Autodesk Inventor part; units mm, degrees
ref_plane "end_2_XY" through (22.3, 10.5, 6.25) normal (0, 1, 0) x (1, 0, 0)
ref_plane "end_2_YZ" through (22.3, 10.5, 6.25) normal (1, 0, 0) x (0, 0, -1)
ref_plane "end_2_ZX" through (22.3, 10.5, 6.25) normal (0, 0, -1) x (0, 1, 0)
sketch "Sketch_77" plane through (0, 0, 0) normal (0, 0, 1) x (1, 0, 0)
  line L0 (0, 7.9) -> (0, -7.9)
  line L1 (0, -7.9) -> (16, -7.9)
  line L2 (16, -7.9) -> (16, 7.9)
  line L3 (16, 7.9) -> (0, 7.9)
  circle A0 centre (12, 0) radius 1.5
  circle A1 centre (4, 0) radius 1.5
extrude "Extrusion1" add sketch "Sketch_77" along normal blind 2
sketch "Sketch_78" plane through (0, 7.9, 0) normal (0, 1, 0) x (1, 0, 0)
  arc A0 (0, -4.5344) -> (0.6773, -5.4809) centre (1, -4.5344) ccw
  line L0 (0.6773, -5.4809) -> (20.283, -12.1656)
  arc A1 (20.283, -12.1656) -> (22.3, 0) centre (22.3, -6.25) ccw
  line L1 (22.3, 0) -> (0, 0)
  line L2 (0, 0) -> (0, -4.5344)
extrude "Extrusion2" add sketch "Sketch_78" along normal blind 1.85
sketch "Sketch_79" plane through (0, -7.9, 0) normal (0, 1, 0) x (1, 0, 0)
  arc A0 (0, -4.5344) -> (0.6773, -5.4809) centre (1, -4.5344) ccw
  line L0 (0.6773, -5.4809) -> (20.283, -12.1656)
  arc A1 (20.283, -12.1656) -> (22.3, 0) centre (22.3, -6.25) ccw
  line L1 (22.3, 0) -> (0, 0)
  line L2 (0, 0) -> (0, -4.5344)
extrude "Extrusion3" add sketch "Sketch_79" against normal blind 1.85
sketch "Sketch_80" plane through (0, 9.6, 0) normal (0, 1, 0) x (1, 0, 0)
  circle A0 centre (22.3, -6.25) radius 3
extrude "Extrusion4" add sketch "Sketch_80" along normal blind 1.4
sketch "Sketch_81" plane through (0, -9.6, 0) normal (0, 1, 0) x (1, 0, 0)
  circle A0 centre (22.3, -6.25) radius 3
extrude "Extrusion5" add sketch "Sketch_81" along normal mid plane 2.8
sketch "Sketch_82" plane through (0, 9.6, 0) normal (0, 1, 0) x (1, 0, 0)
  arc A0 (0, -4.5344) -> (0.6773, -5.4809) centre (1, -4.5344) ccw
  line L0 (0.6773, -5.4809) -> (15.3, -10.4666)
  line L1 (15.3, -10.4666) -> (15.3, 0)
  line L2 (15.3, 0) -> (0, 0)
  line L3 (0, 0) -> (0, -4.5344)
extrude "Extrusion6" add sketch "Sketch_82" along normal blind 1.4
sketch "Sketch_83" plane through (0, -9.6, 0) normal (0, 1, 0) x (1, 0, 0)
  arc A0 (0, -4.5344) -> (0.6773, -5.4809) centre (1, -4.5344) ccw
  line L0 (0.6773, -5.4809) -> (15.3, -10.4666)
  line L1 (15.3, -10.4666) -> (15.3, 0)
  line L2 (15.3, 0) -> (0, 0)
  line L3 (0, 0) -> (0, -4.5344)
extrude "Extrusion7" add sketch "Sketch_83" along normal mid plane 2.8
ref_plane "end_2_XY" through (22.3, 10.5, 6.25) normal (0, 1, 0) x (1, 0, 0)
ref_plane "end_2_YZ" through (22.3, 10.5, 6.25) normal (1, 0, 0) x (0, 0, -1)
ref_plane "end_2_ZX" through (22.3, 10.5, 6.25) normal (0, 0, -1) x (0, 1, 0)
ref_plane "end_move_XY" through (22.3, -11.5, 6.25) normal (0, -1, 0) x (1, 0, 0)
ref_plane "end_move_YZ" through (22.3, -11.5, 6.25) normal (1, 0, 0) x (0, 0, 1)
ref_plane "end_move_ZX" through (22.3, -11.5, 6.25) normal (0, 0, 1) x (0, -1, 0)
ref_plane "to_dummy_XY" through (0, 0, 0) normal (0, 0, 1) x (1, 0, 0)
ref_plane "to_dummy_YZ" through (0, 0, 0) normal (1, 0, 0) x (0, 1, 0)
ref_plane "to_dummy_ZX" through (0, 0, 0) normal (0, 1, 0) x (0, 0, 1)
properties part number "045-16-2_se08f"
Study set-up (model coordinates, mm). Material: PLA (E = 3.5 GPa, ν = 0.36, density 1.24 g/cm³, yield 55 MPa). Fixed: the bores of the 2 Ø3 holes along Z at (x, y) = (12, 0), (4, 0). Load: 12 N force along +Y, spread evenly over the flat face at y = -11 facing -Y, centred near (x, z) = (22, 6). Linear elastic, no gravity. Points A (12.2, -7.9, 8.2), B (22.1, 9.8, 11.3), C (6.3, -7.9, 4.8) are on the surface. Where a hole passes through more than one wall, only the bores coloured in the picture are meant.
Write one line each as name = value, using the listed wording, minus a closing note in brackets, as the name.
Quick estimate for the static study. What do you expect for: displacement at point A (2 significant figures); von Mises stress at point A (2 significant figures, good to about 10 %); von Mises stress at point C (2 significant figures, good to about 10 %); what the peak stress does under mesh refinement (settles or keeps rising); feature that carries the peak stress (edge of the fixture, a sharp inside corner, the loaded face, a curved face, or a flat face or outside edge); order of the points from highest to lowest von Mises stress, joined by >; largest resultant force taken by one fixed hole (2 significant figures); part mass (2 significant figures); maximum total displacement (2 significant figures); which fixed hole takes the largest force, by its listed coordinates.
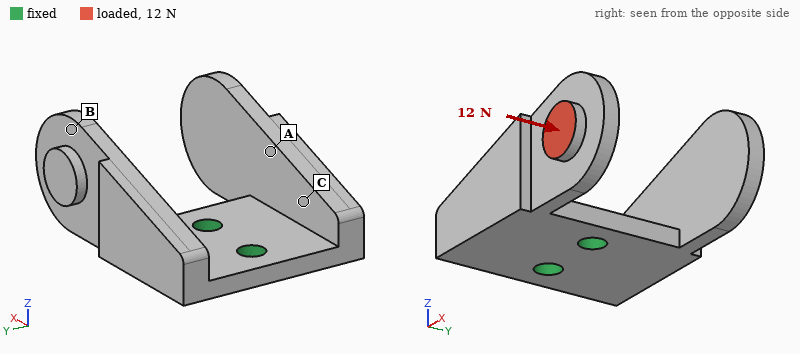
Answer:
displacement at point A = 0.12 mm
von Mises stress at point A = 5.5 MPa
von Mises stress at point C = 3.1 MPa
what the peak stress does under mesh refinement = keeps rising
feature that carries the peak stress = a sharp inside corner
order of the points from highest to lowest von Mises stress, joined by > = A > C > B
largest resultant force taken by one fixed hole = 24 N
part mass = 2.3 g
maximum total displacement = 0.42 mm
which fixed hole takes the largest force, by its listed coordinates = (12, 0)
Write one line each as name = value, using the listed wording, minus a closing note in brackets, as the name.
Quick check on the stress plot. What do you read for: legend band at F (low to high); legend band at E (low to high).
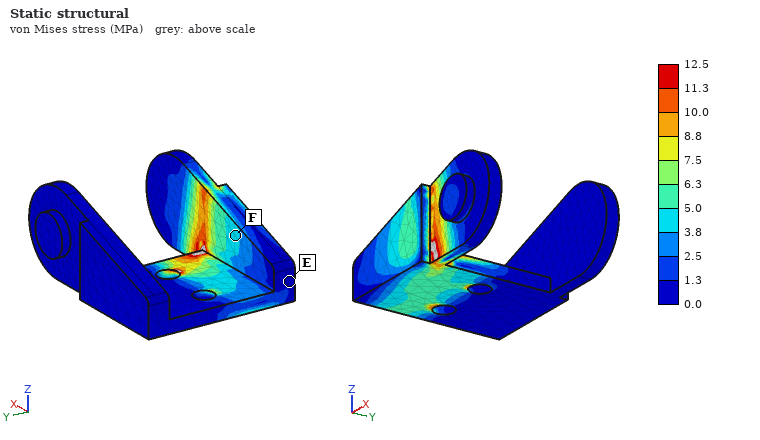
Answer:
legend band at F = 3.8 to 5.0 MPa
legend band at E = 0.0 to 1.3 MPa
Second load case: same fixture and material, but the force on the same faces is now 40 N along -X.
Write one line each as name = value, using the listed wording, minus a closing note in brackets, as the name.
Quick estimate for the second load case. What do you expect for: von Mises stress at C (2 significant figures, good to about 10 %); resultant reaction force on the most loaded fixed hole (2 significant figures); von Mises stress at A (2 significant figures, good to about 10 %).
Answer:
von Mises stress at C = 4.6 MPa
resultant reaction force on the most loaded fixed hole = 51 N
von Mises stress at A = 1.7 MPa
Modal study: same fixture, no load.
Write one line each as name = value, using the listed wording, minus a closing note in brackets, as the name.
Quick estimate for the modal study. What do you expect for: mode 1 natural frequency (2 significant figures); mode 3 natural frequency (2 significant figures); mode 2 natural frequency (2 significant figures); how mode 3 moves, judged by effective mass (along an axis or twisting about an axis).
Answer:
mode 1 natural frequency = 1400 Hz
mode 3 natural frequency = 2200 Hz
mode 2 natural frequency = 1500 Hz
how mode 3 moves, judged by effective mass = along Y
